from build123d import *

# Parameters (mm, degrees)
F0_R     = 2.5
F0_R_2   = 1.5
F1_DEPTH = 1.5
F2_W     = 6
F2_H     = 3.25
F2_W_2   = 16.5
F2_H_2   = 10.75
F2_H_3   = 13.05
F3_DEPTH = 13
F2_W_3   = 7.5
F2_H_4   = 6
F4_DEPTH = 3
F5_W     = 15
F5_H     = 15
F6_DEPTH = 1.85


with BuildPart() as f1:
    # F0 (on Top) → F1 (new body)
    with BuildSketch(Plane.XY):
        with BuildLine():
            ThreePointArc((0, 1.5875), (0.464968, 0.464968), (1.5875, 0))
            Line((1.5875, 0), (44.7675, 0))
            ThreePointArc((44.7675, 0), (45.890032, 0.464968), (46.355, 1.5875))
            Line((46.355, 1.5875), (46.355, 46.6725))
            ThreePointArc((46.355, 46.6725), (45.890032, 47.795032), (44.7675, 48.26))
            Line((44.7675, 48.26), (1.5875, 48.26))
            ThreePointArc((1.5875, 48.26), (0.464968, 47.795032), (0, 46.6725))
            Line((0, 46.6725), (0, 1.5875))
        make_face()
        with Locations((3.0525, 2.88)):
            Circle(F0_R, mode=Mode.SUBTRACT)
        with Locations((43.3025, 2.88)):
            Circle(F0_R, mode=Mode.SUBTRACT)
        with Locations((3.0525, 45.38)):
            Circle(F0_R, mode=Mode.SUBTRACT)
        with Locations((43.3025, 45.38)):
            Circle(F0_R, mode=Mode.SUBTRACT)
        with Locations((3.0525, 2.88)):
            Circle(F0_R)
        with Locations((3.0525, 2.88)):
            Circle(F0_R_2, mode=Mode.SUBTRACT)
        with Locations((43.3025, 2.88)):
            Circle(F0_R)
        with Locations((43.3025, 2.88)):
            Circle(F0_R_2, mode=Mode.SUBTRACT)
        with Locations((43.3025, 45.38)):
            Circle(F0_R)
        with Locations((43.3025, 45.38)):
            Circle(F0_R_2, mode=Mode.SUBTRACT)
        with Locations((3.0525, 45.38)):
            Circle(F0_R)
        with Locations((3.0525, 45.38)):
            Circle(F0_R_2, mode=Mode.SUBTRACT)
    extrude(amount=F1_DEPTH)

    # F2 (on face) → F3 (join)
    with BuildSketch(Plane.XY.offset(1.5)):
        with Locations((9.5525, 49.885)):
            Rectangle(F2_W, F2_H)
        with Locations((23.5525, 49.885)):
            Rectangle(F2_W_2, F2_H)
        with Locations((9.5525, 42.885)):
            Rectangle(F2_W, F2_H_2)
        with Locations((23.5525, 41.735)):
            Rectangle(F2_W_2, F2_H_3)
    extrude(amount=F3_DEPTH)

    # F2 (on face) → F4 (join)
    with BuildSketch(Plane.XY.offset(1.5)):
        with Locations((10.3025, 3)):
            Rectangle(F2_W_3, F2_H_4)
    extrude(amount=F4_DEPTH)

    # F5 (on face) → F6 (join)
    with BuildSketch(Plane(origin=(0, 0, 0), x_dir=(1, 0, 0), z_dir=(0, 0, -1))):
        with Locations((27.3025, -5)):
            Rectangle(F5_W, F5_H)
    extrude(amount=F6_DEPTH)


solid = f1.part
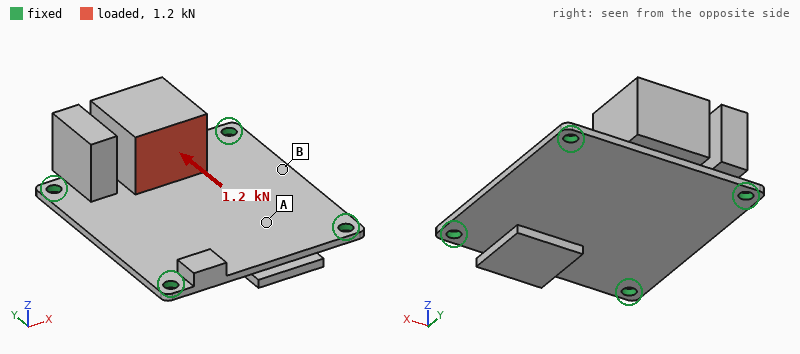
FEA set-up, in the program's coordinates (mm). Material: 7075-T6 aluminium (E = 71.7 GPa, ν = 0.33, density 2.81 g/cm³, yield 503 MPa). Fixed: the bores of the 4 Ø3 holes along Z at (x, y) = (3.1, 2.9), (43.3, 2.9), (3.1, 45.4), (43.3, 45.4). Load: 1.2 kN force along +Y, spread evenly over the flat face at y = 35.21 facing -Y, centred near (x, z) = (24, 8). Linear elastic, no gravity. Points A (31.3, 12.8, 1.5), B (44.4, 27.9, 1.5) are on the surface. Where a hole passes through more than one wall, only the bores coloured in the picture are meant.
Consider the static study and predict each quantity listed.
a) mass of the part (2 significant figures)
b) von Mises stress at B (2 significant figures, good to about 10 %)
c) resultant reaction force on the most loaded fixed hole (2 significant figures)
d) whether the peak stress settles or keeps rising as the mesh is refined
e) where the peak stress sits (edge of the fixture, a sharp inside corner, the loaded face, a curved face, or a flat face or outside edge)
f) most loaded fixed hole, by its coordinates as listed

24 g
81 MPa
470 N
keeps rising
edge of the fixture
(3.1, 45.4)
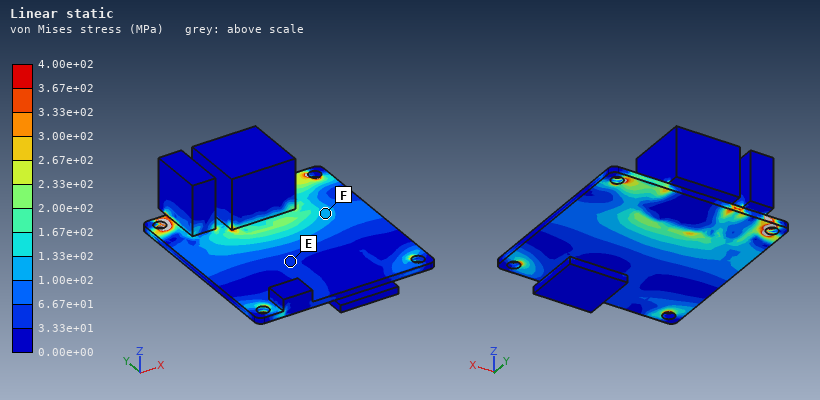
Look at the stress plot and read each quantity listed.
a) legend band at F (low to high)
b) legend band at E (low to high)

1.00e+02 to 1.33e+02 MPa
3.33e+01 to 6.67e+01 MPa
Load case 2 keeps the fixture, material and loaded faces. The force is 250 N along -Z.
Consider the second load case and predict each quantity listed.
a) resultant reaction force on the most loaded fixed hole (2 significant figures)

110 N
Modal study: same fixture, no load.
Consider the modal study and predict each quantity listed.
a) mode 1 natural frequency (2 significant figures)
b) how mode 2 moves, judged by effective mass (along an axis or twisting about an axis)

2300 Hz
along Z
